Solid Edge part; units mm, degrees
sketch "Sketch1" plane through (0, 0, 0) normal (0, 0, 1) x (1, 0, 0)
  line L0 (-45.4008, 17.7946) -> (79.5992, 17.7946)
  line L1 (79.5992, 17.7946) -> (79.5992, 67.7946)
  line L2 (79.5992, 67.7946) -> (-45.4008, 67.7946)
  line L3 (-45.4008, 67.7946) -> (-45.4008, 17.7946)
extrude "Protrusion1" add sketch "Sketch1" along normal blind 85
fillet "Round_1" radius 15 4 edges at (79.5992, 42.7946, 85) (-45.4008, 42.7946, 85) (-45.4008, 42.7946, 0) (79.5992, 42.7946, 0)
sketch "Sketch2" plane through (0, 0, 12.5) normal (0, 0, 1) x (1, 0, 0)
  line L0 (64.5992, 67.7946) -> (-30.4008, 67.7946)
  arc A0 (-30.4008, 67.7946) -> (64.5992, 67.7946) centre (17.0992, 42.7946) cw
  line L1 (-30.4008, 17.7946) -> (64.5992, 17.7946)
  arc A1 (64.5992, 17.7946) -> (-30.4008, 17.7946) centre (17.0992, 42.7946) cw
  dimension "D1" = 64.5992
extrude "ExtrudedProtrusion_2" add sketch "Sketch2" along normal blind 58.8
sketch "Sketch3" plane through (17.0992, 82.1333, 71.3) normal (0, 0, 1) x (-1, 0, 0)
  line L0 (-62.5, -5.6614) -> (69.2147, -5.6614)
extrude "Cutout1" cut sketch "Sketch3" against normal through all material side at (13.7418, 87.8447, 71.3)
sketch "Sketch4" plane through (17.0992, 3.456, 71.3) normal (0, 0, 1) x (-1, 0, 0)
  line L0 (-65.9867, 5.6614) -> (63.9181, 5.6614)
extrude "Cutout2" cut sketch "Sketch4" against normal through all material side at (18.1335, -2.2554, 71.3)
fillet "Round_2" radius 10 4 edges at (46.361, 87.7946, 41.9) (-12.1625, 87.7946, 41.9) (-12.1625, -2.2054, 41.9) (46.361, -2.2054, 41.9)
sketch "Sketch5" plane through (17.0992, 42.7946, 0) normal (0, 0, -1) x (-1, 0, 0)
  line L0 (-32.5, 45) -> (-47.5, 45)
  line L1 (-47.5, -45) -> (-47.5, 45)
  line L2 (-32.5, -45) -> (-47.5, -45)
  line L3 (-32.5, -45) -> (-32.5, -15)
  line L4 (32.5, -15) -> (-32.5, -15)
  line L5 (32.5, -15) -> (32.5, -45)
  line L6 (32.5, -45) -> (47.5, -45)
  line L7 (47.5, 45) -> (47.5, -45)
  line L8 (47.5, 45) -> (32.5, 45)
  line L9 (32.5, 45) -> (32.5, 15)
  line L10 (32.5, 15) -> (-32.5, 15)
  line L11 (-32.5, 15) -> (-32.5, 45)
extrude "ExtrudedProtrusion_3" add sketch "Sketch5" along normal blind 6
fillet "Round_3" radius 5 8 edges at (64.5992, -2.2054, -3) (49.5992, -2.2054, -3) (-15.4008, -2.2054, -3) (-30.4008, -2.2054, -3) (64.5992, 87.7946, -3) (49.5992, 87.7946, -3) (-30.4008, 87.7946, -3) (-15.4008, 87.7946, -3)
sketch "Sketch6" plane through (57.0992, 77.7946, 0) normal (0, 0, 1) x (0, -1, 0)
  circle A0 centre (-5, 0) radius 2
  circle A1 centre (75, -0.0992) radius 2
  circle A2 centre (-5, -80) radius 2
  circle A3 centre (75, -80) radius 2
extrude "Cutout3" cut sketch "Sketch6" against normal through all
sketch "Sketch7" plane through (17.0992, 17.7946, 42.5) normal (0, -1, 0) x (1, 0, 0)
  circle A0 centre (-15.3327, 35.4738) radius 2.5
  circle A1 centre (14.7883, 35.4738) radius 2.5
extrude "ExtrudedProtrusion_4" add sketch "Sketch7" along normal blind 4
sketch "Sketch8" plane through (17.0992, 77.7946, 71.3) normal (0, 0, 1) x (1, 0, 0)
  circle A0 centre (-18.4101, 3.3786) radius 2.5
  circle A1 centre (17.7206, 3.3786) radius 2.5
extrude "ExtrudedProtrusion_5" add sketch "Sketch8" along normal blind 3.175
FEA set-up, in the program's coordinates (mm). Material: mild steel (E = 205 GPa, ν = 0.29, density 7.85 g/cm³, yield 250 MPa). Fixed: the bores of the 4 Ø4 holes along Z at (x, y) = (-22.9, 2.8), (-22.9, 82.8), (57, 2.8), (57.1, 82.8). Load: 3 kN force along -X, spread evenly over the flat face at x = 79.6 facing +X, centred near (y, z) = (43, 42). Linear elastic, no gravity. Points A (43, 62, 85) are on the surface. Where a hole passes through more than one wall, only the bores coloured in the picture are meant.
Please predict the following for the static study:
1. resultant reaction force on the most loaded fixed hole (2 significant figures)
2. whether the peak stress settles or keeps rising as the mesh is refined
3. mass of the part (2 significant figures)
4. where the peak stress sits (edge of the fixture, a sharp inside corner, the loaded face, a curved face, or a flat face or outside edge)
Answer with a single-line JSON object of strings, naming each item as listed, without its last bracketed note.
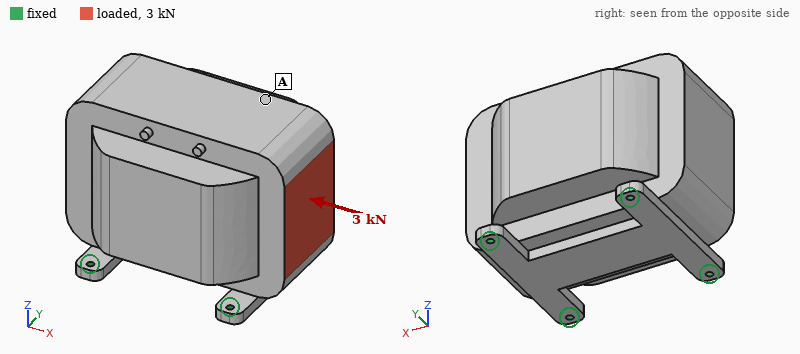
{"resultant reaction force on the most loaded fixed hole": "1.2 kN", "whether the peak stress settles or keeps rising as the mesh is refined": "keeps rising", "mass of the part": "5.8 kg", "where the peak stress sits": "edge of the fixture"}
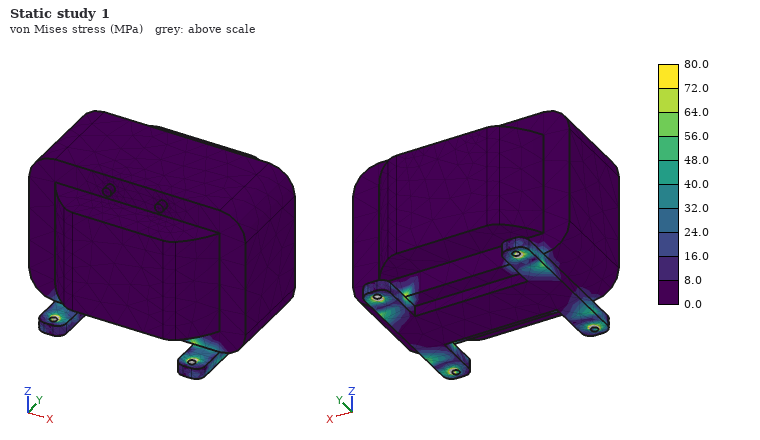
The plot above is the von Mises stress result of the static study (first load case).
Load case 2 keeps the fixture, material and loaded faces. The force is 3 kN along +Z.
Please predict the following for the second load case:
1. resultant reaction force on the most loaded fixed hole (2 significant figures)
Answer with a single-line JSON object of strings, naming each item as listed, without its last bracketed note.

{"resultant reaction force on the most loaded fixed hole": "2.1 kN"}
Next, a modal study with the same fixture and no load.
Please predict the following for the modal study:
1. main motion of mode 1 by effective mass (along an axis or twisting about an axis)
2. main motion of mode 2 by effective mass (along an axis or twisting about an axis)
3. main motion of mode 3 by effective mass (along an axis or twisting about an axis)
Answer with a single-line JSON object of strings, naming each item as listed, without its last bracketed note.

{"main motion of mode 1 by effective mass": "along Y", "main motion of mode 2 by effective mass": "along X", "main motion of mode 3 by effective mass": "along Z"}
